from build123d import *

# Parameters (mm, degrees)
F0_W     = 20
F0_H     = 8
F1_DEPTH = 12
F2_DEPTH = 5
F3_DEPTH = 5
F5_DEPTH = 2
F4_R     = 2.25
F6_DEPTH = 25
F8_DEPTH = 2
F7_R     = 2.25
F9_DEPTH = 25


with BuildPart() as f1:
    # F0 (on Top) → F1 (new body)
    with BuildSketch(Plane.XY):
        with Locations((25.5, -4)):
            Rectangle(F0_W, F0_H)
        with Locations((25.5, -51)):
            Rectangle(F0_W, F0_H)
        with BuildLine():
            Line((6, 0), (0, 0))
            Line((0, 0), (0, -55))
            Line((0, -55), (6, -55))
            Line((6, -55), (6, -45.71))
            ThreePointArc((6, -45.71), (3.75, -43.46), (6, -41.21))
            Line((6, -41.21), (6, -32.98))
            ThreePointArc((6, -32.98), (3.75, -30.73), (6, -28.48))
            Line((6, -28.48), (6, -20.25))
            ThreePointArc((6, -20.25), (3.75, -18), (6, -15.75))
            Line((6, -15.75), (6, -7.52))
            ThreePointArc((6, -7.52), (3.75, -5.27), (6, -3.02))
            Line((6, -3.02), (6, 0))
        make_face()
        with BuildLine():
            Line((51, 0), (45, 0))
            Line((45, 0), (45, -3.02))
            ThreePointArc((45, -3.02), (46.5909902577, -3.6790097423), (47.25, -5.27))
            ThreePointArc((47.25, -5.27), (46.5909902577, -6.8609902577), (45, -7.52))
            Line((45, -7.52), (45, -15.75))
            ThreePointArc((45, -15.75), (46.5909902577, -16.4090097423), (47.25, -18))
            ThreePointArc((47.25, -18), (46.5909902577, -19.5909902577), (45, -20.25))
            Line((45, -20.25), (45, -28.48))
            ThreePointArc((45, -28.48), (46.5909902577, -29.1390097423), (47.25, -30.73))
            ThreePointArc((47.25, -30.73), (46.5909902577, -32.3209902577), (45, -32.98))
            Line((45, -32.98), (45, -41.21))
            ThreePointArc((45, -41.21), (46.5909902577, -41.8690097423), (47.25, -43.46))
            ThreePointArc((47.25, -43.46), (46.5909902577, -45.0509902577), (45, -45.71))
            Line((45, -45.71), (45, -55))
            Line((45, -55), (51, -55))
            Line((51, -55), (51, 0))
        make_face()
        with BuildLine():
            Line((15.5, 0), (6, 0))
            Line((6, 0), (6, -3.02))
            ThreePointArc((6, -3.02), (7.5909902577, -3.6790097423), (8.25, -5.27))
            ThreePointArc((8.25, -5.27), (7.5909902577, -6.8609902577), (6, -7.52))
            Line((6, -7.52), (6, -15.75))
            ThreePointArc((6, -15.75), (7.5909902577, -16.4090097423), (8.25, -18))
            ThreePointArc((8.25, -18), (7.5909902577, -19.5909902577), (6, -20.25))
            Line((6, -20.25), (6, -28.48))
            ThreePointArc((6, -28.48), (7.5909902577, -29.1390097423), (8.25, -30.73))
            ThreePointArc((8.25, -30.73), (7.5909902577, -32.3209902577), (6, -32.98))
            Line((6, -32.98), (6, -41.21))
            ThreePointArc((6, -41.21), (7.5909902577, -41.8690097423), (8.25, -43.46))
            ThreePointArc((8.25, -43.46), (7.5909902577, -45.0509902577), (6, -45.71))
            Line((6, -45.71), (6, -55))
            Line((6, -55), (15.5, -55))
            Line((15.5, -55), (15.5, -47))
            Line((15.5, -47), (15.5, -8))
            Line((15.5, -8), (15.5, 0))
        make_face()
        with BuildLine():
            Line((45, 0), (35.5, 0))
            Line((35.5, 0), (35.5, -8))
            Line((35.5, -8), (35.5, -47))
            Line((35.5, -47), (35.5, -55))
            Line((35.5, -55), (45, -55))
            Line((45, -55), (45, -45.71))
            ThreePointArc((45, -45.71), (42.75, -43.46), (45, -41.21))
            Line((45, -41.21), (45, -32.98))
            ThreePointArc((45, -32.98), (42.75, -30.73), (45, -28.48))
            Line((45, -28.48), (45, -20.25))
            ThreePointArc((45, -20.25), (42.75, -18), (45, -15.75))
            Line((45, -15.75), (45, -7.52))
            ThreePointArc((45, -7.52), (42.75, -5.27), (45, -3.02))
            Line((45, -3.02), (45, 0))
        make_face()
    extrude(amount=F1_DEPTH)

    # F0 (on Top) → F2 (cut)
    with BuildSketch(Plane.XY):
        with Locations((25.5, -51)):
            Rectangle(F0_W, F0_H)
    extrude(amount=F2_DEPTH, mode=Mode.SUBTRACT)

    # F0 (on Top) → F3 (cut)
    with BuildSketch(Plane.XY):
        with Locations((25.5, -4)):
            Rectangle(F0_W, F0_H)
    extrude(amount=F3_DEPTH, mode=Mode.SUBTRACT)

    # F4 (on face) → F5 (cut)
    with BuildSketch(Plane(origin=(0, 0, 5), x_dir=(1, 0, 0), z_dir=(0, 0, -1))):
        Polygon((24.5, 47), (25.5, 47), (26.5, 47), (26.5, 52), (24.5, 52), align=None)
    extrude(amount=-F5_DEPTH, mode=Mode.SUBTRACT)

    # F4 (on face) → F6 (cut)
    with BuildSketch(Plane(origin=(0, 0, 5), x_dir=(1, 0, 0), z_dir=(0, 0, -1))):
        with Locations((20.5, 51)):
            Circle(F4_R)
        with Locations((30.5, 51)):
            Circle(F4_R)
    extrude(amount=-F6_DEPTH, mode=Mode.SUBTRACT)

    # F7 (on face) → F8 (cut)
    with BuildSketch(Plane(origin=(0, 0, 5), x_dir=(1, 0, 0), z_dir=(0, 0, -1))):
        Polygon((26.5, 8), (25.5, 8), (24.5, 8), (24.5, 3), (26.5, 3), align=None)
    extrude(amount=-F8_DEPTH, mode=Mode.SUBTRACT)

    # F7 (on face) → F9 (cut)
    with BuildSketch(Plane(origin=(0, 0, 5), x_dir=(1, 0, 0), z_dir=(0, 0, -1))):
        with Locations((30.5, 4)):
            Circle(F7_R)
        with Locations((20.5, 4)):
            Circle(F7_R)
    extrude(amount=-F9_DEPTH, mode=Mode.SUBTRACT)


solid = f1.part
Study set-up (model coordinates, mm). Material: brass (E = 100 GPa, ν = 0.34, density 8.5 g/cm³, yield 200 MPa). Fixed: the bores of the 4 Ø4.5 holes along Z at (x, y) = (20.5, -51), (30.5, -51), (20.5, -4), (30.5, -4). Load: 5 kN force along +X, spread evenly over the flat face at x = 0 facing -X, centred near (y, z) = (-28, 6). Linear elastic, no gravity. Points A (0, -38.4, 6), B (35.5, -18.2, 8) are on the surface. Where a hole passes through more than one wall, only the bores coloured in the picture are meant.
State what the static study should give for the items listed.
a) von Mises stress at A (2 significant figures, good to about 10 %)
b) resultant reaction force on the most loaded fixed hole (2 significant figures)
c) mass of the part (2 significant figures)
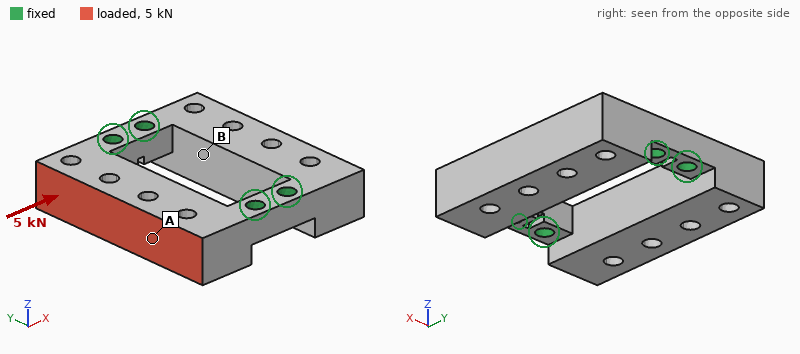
23 MPa
2.6 kN
180 g
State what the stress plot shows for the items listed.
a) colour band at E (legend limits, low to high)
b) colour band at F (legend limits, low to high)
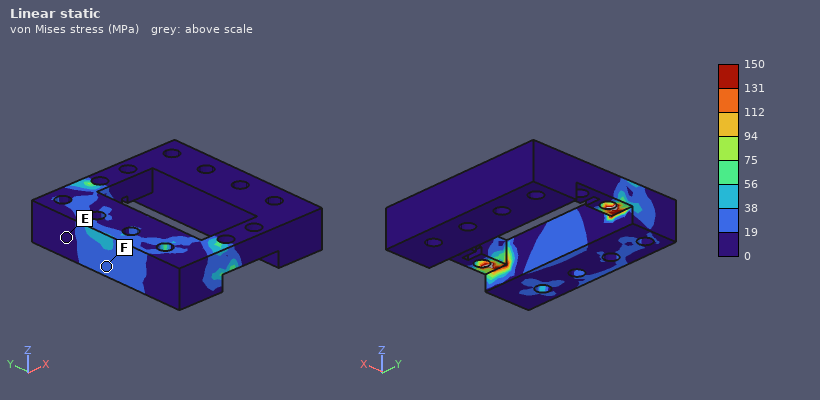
0 to 19 MPa
19 to 38 MPa
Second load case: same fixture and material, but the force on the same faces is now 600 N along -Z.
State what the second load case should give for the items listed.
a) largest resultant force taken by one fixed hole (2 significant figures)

320 N
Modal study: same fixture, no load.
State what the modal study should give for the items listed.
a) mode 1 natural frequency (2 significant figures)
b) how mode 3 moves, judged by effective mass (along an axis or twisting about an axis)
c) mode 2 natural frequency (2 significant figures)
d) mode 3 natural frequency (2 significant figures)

4100 Hz
twisting about X
4100 Hz
9700 Hz
